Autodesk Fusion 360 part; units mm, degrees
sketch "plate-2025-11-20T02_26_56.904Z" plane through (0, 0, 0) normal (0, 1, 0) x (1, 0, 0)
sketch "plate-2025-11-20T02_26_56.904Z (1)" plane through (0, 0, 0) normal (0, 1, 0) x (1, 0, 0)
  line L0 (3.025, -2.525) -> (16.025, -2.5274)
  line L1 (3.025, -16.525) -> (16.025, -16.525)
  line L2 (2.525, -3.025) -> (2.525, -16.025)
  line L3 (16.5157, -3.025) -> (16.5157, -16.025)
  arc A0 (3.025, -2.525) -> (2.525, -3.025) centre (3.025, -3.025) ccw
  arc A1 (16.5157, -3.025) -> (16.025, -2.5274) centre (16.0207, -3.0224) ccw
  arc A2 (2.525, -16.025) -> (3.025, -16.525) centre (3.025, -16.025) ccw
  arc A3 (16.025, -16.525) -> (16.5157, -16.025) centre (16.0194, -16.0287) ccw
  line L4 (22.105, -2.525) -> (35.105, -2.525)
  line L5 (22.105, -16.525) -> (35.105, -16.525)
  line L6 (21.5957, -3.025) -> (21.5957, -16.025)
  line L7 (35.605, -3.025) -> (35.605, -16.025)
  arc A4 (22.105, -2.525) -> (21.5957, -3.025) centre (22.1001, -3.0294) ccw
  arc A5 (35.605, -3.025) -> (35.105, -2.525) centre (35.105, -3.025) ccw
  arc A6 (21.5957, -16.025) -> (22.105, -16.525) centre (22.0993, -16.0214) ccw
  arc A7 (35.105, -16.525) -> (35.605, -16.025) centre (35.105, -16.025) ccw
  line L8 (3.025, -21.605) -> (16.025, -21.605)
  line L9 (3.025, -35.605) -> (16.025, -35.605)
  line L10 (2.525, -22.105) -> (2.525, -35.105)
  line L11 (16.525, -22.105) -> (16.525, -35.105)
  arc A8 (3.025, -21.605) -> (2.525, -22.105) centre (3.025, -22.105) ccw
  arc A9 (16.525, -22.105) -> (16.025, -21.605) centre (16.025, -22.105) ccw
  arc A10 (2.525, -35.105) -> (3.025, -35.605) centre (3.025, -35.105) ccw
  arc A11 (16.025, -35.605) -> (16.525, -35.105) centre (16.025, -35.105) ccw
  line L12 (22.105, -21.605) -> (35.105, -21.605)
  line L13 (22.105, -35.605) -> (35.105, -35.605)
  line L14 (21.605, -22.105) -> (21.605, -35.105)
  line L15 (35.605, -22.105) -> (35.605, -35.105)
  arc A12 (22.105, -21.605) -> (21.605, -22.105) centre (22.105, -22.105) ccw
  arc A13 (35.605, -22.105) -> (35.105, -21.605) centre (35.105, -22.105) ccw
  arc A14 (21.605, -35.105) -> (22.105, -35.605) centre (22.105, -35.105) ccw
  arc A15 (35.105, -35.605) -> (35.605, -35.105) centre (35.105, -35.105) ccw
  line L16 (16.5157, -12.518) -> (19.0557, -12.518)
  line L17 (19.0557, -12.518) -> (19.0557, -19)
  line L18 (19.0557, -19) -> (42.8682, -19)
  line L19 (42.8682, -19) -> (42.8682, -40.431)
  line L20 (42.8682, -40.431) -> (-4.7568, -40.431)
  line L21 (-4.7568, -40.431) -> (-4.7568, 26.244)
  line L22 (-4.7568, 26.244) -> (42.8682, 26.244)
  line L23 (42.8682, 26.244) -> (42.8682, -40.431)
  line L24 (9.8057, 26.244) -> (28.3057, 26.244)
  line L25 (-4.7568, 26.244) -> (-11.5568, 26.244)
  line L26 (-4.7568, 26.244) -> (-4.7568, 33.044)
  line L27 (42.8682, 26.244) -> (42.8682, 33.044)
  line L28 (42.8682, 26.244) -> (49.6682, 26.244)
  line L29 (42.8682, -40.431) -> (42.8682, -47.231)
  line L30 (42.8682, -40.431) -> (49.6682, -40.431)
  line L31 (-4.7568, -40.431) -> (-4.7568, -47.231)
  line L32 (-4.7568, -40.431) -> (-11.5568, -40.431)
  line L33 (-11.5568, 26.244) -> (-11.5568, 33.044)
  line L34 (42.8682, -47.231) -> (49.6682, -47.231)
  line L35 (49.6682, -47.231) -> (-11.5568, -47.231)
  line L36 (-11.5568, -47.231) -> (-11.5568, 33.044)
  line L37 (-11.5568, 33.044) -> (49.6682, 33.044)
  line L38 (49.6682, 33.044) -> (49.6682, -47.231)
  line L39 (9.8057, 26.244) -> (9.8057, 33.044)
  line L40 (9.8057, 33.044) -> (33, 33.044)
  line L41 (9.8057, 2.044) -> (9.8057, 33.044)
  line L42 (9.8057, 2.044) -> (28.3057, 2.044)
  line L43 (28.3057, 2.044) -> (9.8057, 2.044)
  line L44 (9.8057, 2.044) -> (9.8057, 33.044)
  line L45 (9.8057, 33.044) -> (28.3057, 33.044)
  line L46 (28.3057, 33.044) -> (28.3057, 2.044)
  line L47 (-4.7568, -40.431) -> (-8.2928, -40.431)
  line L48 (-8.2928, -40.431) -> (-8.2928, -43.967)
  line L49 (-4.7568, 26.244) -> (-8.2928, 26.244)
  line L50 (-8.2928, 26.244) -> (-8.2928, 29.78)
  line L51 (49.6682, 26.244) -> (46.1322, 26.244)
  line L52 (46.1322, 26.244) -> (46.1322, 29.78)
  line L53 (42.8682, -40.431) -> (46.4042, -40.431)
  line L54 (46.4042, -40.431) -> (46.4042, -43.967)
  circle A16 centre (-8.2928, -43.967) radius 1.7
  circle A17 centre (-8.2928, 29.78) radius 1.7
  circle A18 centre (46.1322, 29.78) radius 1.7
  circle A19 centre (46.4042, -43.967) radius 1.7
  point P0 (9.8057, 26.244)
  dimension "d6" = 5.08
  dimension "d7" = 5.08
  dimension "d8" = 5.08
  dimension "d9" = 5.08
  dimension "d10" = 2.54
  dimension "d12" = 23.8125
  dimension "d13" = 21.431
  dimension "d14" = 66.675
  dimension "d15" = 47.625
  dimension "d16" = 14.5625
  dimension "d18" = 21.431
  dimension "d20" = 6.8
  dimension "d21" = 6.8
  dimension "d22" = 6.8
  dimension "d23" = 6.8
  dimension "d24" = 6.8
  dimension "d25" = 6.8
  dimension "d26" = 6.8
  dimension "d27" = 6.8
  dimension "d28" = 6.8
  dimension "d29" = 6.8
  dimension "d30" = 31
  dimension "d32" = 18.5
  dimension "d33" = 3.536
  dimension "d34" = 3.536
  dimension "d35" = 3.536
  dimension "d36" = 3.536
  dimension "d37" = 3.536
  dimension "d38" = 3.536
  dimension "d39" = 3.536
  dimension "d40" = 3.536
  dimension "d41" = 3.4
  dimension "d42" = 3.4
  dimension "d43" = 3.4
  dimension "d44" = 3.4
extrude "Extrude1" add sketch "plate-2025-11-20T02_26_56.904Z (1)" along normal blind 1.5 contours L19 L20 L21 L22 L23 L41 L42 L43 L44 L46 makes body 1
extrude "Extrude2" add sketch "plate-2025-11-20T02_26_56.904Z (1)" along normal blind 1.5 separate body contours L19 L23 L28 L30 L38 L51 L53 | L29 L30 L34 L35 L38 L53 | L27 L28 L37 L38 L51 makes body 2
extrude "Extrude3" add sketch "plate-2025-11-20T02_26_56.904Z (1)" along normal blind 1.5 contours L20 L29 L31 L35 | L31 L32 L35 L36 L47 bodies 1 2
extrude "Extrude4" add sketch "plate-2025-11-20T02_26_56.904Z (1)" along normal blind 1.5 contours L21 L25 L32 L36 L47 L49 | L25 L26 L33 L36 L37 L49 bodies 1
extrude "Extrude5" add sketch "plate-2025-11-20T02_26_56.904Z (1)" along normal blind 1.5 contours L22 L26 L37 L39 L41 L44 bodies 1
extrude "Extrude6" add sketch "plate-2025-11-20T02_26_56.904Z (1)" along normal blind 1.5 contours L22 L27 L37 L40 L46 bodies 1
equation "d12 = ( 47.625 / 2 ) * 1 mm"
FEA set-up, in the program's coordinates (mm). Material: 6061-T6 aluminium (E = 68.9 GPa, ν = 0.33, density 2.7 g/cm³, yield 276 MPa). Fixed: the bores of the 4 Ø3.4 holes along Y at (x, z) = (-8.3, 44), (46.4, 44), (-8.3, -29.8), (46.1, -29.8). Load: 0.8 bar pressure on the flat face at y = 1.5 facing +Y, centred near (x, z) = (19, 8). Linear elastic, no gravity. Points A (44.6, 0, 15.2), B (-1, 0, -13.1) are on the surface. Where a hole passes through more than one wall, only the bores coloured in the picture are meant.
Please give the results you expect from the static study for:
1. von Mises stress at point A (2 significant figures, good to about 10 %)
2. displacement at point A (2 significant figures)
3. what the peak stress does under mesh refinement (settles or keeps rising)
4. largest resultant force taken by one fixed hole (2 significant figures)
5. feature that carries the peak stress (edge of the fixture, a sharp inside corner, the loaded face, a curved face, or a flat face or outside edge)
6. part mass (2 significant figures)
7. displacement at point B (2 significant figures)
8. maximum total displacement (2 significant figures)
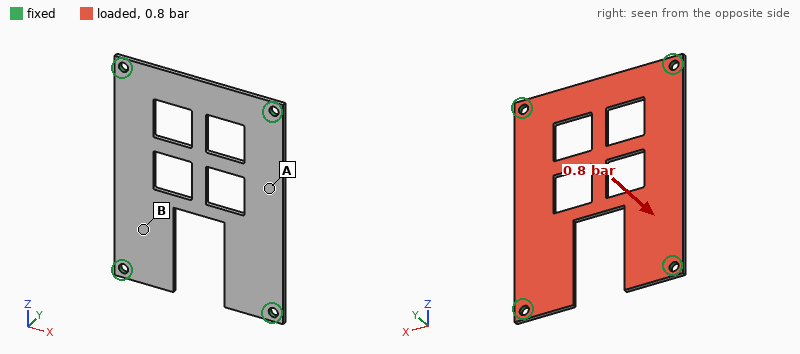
52 MPa
0.36 mm
keeps rising
73 N
edge of the fixture
14 g
0.25 mm
0.57 mm
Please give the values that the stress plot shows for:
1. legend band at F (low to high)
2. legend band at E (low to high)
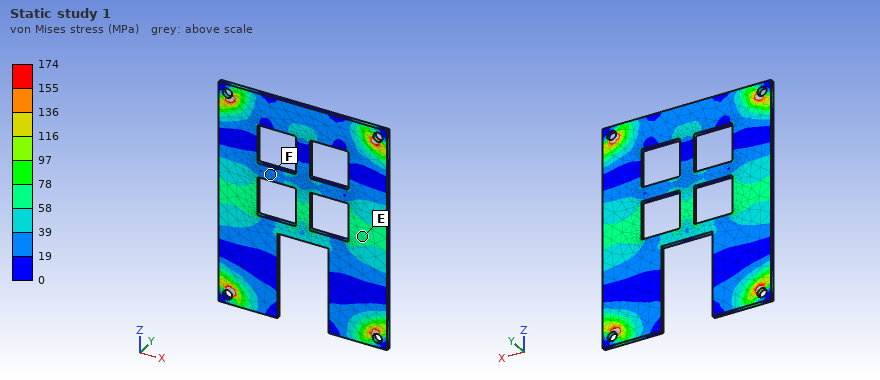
19 to 39 MPa
58 to 78 MPa
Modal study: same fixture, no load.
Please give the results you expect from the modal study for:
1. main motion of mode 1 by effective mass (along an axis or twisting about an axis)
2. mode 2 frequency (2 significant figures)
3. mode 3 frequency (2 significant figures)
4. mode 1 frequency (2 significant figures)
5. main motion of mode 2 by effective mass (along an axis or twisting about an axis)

along Y
1700 Hz
2500 Hz
1200 Hz
twisting about Z
